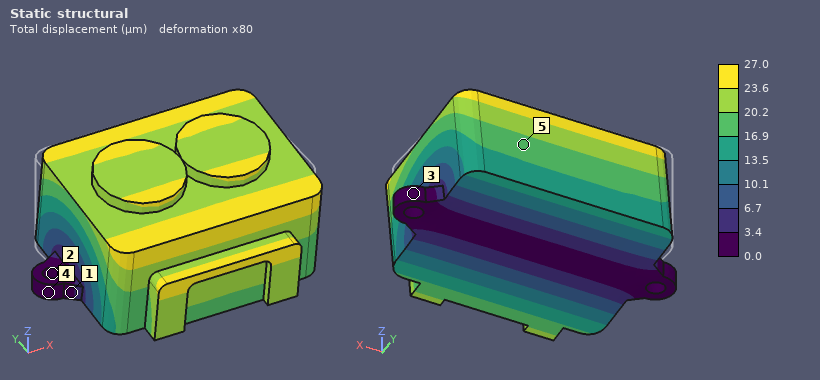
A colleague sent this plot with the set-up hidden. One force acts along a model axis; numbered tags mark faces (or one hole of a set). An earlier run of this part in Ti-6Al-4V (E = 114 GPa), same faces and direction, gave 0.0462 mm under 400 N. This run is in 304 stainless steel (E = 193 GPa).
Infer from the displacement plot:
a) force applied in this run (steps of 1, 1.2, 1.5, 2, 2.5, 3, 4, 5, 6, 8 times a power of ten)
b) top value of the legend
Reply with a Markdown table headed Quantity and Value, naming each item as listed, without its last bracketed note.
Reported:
| Quantity | Value |
|---|---|
| force applied in this run | 400 N |
| top value of the legend | 27.0 µm |
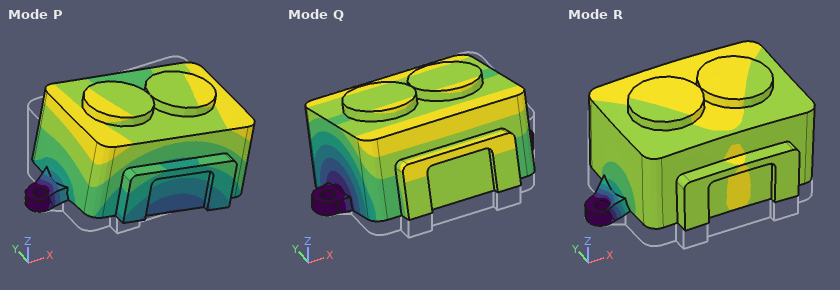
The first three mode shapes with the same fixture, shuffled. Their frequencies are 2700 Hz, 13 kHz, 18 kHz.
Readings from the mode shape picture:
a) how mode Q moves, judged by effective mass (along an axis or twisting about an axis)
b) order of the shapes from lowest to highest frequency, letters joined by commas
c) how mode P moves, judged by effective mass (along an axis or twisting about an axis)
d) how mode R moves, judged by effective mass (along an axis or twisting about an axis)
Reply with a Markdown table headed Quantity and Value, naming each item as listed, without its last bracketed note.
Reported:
| Quantity | Value |
|---|---|
| how mode Q moves, judged by effective mass | along Y |
| order of the shapes from lowest to highest frequency, letters joined by commas | Q, R, P |
| how mode P moves, judged by effective mass | along X |
| how mode R moves, judged by effective mass | along Z |
